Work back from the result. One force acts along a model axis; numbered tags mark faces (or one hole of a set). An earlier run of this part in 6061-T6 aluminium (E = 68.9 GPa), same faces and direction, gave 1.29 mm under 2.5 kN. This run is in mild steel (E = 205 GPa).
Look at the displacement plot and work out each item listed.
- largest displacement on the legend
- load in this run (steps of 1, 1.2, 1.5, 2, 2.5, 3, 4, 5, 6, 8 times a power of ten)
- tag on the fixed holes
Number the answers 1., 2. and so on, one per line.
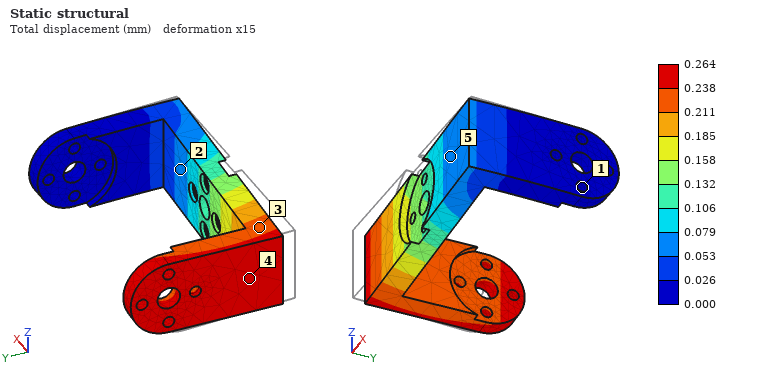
1. 0.264 mm
2. 1.5 kN
3. 1
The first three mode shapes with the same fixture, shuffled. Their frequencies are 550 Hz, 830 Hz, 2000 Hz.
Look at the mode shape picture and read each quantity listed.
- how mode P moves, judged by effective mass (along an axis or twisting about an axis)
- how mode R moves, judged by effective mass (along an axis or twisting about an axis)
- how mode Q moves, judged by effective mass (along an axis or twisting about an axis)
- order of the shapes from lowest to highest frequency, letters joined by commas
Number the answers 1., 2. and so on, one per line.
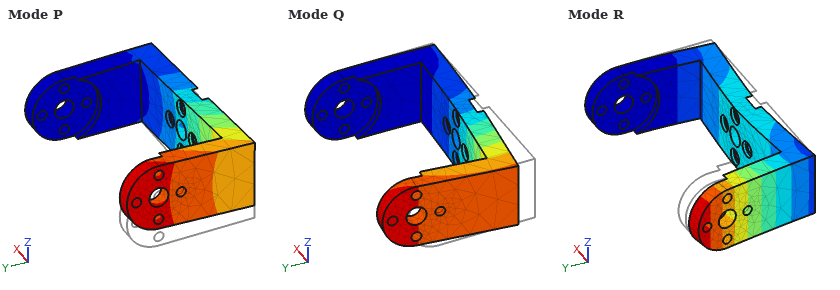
1. along Z
2. along X
3. along Y
4. Q, P, R
